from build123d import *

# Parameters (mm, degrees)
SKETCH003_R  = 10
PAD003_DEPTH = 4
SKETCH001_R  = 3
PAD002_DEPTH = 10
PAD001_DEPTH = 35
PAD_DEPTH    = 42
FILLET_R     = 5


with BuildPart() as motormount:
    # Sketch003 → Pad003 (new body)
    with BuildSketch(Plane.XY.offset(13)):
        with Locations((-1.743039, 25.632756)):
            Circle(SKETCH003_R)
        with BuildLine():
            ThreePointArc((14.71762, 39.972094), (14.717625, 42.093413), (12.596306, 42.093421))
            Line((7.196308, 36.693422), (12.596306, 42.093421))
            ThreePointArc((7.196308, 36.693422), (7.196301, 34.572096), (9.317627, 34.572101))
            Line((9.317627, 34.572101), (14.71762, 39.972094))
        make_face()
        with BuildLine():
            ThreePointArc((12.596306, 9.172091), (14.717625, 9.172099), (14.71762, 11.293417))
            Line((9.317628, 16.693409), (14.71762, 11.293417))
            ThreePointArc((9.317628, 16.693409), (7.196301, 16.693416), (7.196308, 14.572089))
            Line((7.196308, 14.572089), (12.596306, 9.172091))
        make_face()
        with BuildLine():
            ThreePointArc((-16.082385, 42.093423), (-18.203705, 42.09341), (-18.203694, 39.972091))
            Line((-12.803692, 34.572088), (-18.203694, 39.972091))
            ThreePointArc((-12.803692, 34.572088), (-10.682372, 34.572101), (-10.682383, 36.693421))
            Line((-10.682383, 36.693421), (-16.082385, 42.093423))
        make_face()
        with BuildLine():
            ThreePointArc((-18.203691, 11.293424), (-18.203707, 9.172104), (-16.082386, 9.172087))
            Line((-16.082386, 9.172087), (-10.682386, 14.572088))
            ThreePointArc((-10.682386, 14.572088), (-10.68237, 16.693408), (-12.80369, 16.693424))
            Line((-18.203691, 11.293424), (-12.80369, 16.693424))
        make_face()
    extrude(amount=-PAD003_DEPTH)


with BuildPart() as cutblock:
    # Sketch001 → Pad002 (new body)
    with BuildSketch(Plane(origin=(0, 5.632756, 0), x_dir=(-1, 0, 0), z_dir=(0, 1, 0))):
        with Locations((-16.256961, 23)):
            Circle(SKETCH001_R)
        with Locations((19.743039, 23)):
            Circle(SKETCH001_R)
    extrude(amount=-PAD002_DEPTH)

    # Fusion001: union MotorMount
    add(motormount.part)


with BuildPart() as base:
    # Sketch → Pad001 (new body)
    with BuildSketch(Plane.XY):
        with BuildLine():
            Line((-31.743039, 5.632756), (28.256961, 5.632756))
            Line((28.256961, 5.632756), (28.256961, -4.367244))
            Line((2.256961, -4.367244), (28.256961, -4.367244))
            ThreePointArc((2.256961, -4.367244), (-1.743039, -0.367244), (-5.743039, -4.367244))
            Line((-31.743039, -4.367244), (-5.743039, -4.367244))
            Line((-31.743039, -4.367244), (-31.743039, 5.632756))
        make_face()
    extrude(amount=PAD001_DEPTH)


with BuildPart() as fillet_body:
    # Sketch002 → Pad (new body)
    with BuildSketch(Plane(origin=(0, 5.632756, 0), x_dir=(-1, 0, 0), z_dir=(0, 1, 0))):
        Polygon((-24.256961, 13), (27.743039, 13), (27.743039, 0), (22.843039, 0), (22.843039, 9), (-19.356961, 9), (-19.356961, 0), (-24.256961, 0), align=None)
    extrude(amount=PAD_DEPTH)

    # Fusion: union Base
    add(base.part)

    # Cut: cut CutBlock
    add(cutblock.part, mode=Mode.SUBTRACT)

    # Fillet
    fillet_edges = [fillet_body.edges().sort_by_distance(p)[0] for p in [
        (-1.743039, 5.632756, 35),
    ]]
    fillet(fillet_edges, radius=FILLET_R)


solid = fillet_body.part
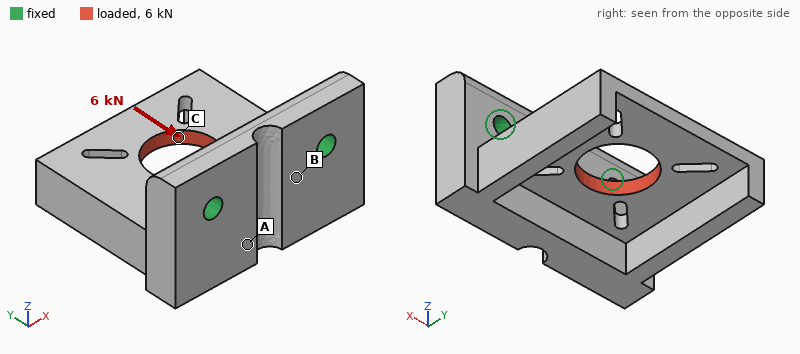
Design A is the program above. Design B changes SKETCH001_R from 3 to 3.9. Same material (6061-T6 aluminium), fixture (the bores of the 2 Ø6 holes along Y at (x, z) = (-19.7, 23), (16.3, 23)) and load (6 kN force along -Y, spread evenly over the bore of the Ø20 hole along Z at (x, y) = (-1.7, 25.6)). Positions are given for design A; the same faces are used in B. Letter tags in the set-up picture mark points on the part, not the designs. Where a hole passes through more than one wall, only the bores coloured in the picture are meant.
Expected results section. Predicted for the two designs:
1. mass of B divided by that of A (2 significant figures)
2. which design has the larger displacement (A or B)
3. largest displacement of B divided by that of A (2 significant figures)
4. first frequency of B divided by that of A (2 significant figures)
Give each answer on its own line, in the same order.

0.99
A
0.81
1.0
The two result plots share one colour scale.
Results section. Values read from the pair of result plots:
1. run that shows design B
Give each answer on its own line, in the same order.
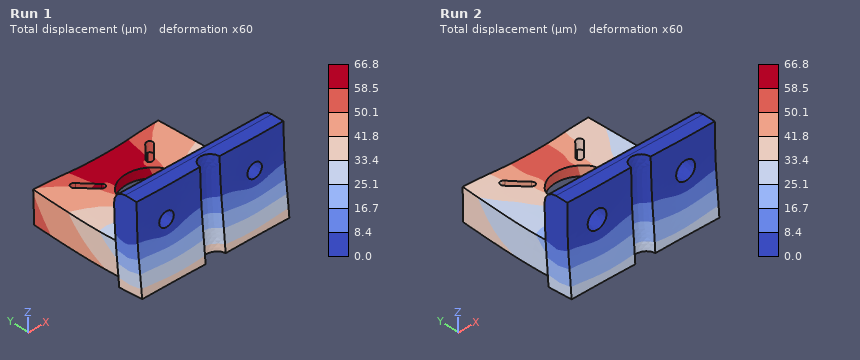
Run 2
